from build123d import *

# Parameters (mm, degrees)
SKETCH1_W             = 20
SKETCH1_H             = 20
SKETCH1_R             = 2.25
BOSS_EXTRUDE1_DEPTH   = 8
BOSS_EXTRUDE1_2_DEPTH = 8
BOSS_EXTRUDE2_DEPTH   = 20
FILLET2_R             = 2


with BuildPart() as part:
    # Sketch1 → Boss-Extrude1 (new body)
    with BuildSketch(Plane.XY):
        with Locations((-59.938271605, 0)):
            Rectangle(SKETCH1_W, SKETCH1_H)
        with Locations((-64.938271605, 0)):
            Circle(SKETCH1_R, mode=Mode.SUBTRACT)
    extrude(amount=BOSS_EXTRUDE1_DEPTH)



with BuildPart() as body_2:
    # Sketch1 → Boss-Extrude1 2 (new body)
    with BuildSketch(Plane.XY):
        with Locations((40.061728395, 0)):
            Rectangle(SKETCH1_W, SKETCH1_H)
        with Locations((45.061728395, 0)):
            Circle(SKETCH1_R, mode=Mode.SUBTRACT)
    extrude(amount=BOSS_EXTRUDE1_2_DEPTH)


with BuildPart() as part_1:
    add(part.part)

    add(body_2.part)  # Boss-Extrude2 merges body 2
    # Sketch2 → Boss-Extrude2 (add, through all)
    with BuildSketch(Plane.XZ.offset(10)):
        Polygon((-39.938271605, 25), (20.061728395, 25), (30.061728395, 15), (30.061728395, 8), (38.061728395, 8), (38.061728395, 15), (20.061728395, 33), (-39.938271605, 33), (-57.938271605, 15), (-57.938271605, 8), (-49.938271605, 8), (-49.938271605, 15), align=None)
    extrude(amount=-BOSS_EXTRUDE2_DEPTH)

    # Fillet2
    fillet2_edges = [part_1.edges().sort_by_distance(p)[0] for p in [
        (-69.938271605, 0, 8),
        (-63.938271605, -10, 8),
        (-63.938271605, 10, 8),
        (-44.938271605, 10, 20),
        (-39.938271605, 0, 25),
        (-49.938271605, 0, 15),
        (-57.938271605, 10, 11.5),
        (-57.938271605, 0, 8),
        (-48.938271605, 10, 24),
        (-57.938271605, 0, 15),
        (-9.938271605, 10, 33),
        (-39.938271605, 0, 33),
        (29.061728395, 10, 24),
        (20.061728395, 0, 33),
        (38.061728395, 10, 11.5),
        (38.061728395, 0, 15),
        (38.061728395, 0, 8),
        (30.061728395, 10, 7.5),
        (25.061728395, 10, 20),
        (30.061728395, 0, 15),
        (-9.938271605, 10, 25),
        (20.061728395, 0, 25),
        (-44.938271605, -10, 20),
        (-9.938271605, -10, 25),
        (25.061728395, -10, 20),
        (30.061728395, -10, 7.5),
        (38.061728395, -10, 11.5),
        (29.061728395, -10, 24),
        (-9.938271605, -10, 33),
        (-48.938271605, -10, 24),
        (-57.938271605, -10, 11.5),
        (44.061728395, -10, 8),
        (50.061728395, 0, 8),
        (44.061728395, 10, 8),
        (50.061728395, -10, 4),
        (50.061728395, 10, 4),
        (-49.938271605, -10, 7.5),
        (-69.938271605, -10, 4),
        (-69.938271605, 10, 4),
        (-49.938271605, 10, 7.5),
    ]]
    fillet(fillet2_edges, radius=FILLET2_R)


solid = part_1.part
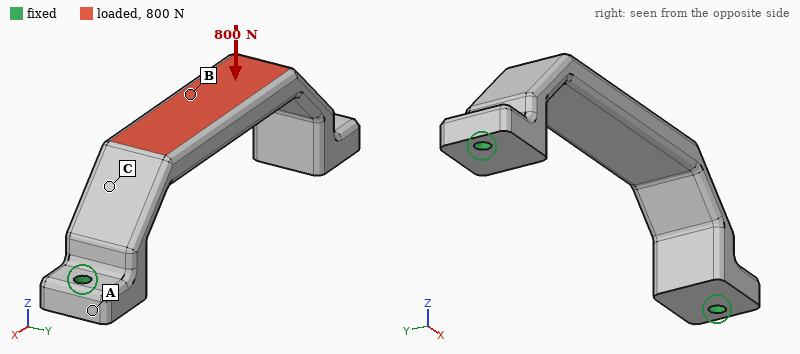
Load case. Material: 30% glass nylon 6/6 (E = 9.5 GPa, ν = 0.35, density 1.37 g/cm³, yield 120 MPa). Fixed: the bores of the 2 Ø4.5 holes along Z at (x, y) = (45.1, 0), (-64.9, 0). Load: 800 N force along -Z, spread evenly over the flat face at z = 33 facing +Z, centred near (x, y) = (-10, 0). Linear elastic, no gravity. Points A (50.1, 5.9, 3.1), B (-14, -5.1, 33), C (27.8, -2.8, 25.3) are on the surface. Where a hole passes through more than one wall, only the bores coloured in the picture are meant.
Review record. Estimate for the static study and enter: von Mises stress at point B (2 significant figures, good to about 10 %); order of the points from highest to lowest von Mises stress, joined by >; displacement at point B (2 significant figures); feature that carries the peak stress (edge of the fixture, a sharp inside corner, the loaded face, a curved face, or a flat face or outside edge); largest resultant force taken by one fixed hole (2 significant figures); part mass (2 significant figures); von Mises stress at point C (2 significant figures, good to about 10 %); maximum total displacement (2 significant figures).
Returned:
22 MPa
B > C > A
0.23 mm
a curved face
610 N
30 g
10 MPa
0.25 mm
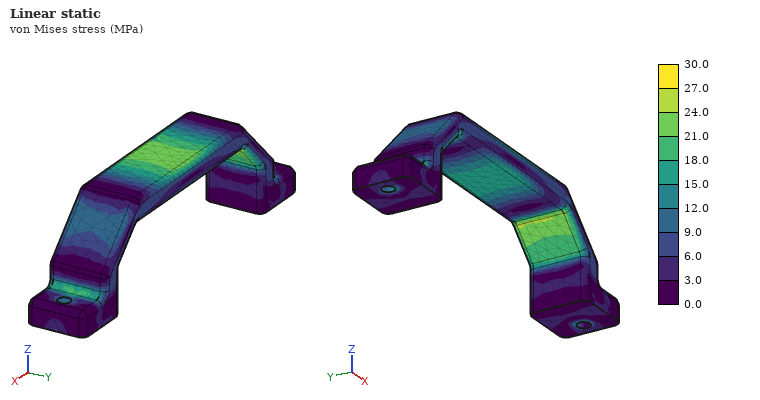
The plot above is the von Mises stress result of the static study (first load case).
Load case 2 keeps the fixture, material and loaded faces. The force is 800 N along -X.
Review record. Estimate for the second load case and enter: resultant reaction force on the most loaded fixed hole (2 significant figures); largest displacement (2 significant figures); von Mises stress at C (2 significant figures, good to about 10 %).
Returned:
430 N
0.19 mm
9.8 MPa
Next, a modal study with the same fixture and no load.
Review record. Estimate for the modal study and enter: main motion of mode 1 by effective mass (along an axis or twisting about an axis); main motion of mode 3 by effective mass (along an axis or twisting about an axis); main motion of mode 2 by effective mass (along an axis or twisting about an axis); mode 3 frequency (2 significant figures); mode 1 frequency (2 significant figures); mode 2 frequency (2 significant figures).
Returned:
along Y
along Z
along X
2900 Hz
1600 Hz
2300 Hz
